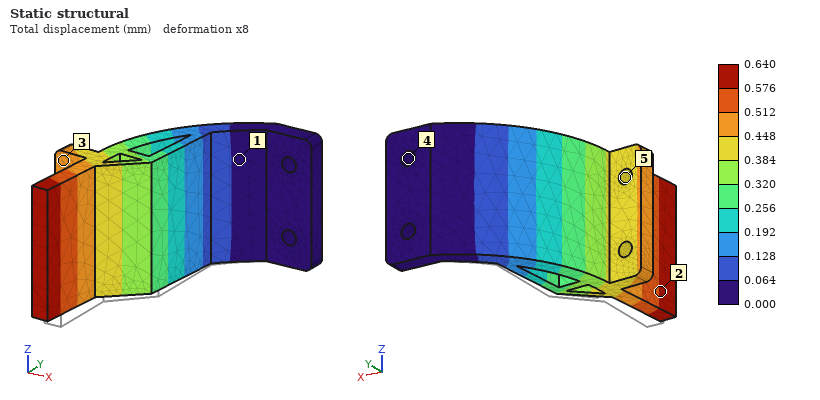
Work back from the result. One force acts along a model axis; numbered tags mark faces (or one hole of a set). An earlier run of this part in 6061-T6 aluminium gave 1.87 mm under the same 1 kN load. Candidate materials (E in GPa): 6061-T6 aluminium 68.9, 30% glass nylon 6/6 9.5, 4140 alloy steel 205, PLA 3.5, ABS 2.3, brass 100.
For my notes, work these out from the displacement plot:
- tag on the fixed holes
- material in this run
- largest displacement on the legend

4
4140 alloy steel
0.640 mm
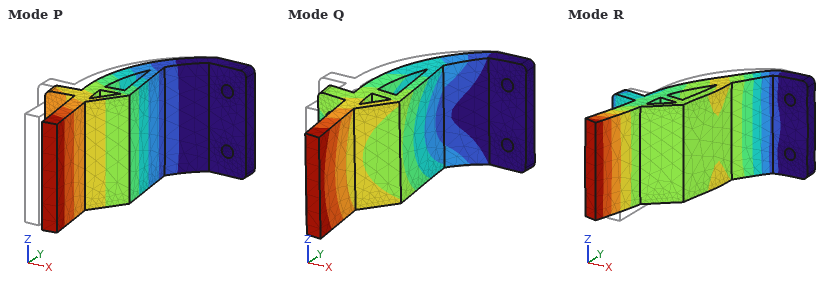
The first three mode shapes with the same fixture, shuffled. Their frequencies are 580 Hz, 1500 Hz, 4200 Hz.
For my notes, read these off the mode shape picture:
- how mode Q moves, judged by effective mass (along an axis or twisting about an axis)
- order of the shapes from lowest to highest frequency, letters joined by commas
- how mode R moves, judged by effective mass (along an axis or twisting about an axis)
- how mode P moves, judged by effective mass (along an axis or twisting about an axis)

along Z
P, Q, R
along Y
along X
